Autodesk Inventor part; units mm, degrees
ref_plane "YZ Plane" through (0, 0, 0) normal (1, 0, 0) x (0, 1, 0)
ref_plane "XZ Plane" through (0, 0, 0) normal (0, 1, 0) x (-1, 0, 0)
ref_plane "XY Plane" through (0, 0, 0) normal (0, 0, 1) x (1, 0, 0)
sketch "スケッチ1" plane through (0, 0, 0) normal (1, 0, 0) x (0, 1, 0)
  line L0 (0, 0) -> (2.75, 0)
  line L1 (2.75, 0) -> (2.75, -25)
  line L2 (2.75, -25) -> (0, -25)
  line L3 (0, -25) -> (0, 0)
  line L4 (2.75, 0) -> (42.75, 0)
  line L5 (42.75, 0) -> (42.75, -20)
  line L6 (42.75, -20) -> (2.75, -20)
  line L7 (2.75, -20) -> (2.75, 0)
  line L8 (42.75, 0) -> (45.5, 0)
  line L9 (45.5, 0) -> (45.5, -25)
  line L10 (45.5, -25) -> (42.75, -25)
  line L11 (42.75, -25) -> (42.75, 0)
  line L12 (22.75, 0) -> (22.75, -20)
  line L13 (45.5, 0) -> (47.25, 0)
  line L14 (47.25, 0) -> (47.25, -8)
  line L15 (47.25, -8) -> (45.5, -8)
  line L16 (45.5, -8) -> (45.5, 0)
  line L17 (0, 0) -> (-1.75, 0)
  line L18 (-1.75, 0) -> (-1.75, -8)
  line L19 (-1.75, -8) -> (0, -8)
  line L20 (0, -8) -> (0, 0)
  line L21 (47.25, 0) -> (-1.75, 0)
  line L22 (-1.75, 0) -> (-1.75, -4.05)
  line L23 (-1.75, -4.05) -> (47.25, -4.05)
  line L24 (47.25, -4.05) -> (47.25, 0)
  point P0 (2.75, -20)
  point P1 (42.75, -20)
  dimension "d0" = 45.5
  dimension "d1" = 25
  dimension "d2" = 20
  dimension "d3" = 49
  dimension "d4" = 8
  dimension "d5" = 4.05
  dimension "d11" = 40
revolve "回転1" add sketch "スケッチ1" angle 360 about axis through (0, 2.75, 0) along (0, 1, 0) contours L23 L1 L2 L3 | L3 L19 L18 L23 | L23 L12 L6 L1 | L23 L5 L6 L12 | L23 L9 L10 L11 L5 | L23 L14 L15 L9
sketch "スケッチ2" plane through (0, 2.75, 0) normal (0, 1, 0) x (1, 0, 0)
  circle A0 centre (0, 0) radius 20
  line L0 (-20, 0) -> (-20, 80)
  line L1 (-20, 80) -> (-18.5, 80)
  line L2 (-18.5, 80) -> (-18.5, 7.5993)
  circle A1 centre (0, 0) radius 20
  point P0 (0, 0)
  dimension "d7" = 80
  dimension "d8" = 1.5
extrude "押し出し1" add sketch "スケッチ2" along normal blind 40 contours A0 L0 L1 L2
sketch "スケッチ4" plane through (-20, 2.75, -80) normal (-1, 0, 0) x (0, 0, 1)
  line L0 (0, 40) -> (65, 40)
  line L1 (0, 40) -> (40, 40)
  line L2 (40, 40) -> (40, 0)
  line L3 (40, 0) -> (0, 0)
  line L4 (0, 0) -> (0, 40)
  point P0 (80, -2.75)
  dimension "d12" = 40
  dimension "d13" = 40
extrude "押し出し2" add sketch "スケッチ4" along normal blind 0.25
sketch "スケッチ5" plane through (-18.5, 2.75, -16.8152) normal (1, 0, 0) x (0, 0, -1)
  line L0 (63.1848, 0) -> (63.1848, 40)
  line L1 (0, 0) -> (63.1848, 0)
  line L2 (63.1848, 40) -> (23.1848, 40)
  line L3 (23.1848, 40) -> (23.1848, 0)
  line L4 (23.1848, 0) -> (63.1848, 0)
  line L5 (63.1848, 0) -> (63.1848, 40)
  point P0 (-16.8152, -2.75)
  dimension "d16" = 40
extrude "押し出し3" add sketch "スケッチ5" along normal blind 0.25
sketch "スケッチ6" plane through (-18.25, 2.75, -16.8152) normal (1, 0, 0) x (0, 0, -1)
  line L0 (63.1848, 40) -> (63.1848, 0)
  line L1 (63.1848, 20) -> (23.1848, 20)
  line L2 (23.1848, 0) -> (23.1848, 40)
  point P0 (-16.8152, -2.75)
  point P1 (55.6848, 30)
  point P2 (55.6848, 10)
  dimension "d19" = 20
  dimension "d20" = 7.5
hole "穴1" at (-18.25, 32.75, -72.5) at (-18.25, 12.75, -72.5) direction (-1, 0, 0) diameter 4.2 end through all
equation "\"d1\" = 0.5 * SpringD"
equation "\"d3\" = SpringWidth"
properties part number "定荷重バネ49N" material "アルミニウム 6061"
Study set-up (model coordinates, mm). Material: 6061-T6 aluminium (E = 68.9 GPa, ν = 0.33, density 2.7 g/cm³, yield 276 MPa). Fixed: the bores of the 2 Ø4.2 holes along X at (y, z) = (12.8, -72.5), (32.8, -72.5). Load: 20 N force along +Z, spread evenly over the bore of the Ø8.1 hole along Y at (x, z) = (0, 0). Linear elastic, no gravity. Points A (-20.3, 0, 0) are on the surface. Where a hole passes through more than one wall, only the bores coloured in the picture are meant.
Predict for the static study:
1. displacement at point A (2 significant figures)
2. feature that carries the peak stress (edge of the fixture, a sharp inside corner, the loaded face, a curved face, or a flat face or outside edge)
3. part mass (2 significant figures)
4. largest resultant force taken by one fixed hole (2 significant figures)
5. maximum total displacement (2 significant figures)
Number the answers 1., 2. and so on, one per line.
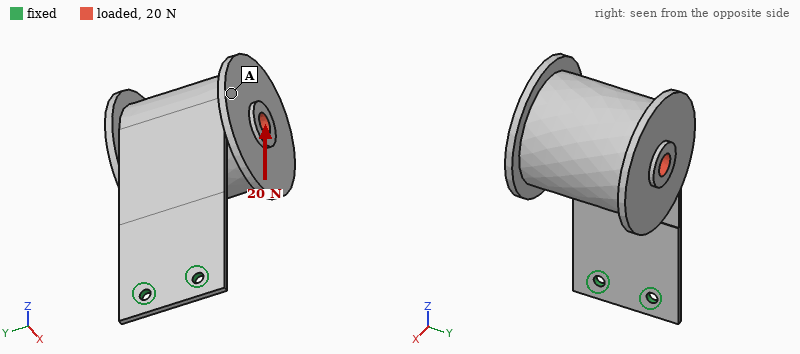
1. 0.71 mm
2. a flat face or outside edge
3. 170 g
4. 10 N
5. 1.3 mm
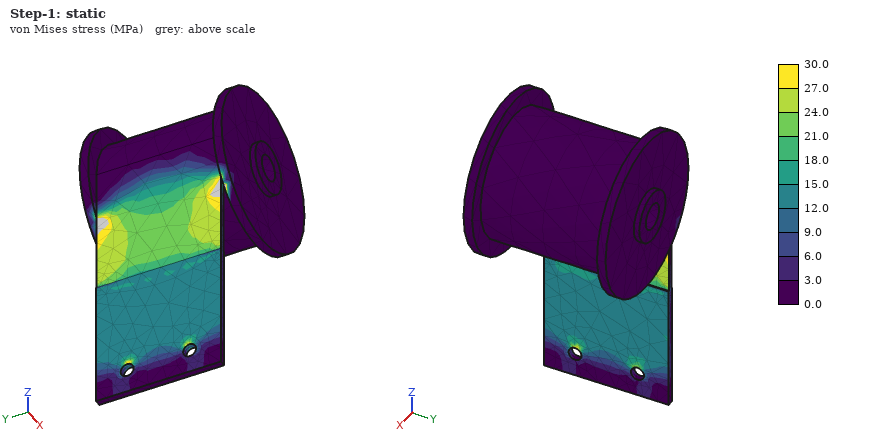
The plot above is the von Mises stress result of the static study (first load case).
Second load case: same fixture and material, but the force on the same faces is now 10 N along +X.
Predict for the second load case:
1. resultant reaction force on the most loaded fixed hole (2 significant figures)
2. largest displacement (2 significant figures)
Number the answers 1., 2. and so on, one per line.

1. 5.0 N
2. 1.3 mm
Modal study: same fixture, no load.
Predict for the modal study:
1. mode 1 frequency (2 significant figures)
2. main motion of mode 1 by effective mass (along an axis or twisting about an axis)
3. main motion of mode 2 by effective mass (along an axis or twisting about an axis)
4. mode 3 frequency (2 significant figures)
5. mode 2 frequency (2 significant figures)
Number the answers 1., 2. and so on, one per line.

1. 38 Hz
2. along X
3. along Y
4. 190 Hz
5. 100 Hz
